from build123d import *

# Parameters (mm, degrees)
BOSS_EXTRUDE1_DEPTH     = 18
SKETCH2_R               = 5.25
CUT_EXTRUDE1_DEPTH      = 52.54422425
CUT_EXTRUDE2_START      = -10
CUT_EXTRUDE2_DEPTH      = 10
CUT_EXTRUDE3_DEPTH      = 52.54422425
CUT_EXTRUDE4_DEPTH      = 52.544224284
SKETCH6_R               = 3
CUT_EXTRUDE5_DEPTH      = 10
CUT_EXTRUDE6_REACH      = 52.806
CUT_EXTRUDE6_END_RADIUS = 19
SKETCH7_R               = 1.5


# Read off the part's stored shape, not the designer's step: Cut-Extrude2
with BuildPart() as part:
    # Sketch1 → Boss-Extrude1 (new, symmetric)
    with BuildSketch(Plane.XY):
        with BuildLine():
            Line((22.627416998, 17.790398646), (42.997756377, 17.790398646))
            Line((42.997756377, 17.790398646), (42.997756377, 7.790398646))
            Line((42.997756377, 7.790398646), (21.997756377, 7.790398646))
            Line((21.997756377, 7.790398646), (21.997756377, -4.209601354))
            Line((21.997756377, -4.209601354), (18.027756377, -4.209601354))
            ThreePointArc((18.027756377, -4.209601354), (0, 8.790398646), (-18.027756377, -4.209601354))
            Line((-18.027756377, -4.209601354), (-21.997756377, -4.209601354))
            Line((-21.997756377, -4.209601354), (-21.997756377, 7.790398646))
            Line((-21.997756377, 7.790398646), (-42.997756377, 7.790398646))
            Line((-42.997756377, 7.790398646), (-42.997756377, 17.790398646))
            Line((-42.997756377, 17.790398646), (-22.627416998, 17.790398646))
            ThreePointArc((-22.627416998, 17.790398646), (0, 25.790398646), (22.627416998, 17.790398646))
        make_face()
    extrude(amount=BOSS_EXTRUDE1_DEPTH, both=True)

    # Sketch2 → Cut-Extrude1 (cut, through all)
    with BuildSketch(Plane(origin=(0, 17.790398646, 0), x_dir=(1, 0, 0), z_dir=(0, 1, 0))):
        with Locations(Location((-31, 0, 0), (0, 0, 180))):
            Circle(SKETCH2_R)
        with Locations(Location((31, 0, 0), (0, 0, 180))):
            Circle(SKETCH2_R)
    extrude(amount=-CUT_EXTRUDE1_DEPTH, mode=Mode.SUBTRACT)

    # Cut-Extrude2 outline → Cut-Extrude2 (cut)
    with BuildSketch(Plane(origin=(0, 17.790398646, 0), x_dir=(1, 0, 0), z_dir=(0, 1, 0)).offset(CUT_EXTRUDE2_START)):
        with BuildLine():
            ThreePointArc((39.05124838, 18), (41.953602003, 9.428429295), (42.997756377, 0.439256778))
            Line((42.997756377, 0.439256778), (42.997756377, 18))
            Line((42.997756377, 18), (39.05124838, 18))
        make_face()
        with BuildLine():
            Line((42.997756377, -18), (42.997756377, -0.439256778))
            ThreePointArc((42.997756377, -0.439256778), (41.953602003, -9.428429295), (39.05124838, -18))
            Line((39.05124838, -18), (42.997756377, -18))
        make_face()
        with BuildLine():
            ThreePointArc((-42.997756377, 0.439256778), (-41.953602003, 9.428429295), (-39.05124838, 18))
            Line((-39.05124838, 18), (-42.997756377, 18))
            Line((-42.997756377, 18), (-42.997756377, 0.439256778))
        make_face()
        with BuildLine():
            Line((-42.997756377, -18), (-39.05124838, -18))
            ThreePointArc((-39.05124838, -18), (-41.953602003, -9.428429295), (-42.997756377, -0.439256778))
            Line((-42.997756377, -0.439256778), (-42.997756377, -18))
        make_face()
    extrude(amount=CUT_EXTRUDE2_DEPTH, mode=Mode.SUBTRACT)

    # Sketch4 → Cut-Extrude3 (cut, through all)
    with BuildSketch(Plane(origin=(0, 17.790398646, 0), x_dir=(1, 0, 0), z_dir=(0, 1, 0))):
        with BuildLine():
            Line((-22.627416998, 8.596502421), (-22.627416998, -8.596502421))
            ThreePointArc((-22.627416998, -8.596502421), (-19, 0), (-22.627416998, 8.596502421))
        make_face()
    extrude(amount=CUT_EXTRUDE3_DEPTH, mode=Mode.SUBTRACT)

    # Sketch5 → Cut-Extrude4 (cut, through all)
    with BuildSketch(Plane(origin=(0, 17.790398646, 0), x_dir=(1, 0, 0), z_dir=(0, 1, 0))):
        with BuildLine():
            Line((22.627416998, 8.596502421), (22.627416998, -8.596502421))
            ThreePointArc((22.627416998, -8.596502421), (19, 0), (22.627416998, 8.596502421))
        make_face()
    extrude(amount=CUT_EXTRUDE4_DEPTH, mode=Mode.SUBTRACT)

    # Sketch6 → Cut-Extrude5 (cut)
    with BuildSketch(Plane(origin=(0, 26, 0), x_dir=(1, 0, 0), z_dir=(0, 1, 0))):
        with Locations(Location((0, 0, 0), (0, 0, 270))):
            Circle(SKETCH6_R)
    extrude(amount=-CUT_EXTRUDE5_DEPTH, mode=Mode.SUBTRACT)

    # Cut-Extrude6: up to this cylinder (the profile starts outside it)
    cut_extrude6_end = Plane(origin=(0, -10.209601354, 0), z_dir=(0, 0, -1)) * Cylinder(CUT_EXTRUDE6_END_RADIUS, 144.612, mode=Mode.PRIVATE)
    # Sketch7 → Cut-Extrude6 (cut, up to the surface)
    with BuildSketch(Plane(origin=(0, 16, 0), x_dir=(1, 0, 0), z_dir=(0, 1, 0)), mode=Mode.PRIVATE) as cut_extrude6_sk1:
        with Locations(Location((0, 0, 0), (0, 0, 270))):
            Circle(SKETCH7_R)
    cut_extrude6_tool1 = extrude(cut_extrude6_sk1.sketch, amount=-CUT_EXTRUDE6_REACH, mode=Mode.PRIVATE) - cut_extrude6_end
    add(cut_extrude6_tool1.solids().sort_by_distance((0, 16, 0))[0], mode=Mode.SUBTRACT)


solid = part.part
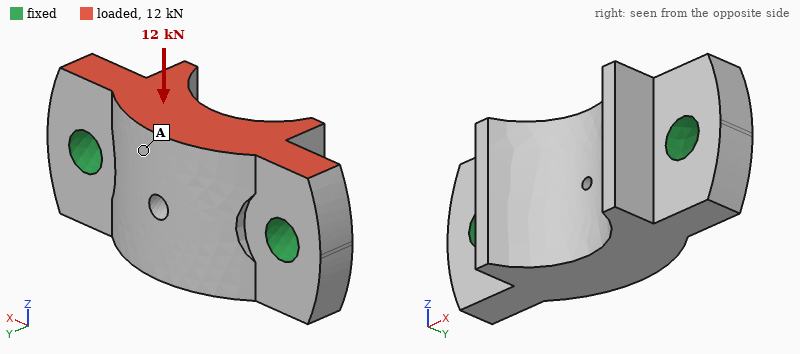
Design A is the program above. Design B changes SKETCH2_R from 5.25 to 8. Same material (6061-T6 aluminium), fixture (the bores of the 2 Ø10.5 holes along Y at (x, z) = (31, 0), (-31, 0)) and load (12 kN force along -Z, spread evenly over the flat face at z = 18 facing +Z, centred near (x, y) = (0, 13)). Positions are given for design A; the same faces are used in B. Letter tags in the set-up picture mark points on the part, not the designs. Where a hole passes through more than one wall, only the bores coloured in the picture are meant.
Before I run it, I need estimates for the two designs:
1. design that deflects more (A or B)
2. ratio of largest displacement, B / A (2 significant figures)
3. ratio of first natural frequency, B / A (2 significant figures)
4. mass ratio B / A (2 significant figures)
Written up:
A
0.75
1.3
0.95
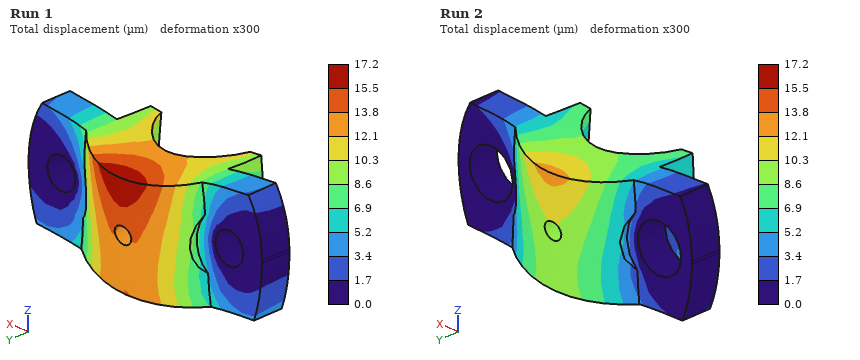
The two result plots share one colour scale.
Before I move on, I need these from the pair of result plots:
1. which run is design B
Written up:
Run 2
